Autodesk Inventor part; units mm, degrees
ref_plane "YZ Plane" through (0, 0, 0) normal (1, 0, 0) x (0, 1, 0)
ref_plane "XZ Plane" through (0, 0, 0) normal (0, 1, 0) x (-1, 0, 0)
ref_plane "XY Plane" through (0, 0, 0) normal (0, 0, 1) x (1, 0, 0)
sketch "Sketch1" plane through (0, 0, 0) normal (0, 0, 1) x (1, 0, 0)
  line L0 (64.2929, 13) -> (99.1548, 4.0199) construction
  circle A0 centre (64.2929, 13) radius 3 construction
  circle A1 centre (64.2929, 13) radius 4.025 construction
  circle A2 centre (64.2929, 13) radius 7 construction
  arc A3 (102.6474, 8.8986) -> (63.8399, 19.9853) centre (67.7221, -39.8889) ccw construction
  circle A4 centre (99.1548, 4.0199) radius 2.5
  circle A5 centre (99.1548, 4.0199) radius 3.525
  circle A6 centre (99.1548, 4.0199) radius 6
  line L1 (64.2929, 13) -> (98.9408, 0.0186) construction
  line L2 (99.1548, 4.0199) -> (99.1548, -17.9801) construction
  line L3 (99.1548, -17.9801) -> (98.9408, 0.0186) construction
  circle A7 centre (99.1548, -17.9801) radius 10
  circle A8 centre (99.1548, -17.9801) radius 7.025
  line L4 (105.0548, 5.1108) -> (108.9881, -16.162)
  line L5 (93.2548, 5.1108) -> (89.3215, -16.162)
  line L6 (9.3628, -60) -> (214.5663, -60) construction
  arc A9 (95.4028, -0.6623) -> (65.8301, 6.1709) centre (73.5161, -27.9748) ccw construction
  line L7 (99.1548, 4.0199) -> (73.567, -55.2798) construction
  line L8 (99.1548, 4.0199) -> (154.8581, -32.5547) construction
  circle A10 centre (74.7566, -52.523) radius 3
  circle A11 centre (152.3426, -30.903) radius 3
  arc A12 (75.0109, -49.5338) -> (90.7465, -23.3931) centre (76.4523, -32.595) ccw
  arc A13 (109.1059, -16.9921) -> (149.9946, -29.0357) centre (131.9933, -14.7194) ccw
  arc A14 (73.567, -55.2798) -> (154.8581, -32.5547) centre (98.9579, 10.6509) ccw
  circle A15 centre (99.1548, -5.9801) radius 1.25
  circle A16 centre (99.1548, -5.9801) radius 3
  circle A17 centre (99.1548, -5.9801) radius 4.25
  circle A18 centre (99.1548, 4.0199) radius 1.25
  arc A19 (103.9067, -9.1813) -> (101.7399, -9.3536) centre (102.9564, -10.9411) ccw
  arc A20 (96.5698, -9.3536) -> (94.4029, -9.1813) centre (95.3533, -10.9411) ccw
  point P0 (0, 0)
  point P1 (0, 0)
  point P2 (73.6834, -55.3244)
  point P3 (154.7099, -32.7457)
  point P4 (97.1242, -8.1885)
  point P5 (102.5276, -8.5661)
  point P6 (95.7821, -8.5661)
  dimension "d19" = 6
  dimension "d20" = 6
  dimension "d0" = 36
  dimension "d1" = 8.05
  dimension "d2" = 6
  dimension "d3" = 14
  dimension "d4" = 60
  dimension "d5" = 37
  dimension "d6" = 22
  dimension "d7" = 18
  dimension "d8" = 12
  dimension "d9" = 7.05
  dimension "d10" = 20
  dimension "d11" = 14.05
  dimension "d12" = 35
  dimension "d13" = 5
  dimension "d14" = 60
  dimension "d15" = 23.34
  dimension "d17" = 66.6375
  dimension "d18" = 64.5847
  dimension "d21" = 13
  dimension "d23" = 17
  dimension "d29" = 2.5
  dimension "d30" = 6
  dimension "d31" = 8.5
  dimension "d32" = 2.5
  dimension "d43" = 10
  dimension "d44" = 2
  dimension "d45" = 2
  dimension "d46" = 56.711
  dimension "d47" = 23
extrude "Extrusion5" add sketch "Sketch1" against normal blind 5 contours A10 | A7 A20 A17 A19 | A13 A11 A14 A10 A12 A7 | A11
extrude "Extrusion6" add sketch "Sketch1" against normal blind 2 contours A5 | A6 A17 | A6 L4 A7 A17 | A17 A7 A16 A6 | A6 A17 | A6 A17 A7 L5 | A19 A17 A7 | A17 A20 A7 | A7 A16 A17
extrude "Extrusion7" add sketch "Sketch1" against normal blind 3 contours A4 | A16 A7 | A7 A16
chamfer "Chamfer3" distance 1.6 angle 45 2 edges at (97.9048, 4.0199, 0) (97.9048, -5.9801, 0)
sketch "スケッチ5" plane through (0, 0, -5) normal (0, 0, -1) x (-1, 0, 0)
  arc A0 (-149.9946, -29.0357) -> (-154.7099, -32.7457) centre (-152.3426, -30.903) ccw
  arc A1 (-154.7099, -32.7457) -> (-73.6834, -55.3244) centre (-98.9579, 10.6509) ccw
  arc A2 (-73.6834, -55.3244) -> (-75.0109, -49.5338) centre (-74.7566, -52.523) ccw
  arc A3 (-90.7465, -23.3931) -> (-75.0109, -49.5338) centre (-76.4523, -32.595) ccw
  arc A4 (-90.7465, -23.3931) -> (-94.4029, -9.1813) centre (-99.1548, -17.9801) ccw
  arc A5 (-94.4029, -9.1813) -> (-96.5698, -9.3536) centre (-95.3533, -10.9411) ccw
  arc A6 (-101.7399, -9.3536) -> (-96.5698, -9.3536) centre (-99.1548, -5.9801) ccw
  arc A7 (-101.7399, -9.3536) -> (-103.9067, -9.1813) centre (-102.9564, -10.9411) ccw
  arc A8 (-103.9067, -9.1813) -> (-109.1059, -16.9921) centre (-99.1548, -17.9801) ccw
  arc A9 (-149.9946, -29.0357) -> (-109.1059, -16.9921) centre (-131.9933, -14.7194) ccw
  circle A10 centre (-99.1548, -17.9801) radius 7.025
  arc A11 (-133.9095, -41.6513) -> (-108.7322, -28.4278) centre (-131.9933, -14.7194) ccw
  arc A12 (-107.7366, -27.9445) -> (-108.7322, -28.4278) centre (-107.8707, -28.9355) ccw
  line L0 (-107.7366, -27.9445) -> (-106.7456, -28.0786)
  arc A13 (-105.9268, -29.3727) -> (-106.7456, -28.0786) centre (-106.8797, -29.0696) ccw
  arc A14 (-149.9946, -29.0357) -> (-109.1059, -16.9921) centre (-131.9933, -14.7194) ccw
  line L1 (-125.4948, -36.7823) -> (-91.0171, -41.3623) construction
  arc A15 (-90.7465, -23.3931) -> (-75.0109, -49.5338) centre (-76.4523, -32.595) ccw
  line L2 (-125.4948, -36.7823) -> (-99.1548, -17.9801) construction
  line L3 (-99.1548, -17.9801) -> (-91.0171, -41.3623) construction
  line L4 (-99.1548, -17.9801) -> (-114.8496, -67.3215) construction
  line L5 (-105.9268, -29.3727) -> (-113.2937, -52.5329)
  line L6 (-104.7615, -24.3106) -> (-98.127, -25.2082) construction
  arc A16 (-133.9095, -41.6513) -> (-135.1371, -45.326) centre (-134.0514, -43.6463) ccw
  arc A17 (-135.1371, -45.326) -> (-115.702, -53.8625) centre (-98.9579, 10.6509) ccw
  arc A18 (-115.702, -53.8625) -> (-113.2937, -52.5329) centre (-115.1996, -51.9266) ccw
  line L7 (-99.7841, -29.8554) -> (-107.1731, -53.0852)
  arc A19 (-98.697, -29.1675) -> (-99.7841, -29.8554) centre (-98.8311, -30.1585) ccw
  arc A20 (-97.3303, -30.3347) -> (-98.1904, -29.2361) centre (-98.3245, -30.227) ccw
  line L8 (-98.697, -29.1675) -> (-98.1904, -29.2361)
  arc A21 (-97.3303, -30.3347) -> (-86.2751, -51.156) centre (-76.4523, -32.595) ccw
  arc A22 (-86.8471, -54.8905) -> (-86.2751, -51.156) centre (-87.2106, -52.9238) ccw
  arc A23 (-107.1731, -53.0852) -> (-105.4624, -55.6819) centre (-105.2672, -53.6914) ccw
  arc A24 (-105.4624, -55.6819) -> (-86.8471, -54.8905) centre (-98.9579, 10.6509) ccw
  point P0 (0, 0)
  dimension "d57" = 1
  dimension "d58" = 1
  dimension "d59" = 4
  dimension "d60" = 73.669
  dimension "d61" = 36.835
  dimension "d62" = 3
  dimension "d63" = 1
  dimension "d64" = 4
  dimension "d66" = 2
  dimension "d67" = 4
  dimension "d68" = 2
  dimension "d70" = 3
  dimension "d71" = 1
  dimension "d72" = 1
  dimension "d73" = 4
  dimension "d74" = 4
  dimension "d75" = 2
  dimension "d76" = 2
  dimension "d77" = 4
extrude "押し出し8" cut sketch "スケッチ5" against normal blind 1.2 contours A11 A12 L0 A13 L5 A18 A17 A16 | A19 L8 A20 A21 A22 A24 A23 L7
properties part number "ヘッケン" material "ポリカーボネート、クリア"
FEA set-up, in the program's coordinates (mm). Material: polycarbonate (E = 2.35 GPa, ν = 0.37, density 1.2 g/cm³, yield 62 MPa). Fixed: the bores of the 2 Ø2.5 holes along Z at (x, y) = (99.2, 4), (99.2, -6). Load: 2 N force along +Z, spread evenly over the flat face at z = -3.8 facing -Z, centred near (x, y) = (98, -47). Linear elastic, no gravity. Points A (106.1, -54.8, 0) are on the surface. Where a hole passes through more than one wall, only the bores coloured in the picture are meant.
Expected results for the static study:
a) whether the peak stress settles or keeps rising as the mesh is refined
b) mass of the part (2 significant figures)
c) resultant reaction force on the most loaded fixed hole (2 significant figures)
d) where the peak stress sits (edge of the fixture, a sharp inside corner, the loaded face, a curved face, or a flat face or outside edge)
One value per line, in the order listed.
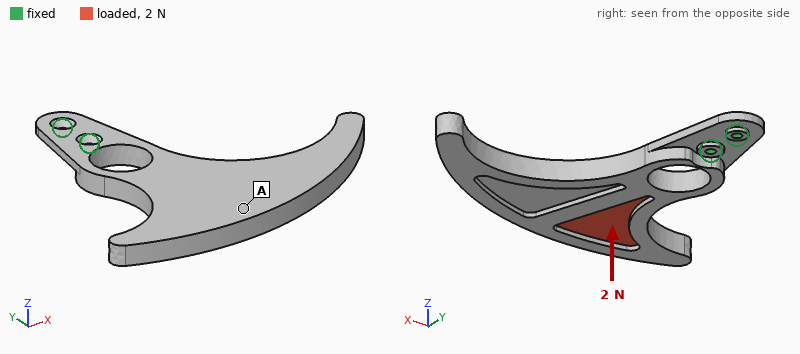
keeps rising
9.8 g
12 N
edge of the fixture
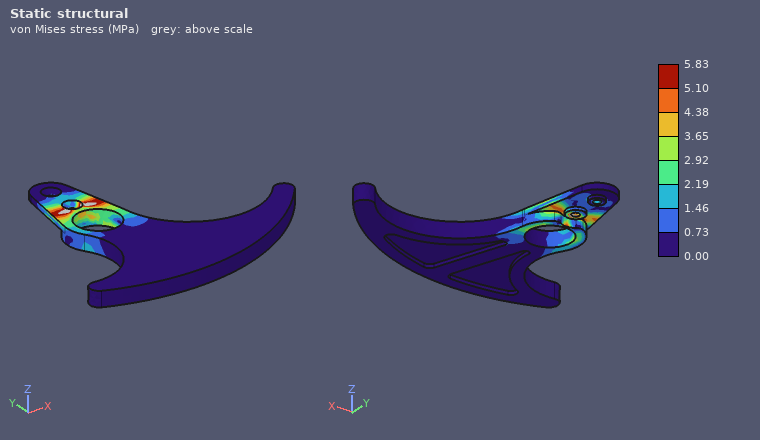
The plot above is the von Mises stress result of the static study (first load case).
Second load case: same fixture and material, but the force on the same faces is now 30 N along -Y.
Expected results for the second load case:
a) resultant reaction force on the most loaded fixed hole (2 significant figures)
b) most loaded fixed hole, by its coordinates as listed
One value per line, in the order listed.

28 N
(99.2, -6)
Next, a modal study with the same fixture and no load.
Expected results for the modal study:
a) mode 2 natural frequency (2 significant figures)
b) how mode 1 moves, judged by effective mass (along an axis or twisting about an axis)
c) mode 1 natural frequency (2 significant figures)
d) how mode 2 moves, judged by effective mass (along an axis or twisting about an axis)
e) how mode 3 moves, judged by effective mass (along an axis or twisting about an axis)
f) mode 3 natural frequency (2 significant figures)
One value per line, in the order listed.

160 Hz
along Z
85 Hz
twisting about Y
along X
300 Hz
